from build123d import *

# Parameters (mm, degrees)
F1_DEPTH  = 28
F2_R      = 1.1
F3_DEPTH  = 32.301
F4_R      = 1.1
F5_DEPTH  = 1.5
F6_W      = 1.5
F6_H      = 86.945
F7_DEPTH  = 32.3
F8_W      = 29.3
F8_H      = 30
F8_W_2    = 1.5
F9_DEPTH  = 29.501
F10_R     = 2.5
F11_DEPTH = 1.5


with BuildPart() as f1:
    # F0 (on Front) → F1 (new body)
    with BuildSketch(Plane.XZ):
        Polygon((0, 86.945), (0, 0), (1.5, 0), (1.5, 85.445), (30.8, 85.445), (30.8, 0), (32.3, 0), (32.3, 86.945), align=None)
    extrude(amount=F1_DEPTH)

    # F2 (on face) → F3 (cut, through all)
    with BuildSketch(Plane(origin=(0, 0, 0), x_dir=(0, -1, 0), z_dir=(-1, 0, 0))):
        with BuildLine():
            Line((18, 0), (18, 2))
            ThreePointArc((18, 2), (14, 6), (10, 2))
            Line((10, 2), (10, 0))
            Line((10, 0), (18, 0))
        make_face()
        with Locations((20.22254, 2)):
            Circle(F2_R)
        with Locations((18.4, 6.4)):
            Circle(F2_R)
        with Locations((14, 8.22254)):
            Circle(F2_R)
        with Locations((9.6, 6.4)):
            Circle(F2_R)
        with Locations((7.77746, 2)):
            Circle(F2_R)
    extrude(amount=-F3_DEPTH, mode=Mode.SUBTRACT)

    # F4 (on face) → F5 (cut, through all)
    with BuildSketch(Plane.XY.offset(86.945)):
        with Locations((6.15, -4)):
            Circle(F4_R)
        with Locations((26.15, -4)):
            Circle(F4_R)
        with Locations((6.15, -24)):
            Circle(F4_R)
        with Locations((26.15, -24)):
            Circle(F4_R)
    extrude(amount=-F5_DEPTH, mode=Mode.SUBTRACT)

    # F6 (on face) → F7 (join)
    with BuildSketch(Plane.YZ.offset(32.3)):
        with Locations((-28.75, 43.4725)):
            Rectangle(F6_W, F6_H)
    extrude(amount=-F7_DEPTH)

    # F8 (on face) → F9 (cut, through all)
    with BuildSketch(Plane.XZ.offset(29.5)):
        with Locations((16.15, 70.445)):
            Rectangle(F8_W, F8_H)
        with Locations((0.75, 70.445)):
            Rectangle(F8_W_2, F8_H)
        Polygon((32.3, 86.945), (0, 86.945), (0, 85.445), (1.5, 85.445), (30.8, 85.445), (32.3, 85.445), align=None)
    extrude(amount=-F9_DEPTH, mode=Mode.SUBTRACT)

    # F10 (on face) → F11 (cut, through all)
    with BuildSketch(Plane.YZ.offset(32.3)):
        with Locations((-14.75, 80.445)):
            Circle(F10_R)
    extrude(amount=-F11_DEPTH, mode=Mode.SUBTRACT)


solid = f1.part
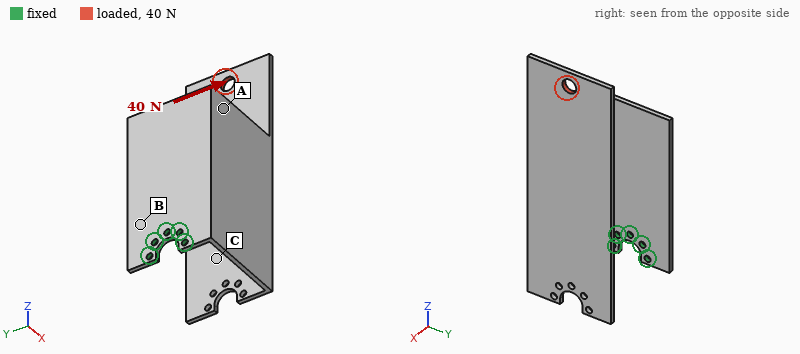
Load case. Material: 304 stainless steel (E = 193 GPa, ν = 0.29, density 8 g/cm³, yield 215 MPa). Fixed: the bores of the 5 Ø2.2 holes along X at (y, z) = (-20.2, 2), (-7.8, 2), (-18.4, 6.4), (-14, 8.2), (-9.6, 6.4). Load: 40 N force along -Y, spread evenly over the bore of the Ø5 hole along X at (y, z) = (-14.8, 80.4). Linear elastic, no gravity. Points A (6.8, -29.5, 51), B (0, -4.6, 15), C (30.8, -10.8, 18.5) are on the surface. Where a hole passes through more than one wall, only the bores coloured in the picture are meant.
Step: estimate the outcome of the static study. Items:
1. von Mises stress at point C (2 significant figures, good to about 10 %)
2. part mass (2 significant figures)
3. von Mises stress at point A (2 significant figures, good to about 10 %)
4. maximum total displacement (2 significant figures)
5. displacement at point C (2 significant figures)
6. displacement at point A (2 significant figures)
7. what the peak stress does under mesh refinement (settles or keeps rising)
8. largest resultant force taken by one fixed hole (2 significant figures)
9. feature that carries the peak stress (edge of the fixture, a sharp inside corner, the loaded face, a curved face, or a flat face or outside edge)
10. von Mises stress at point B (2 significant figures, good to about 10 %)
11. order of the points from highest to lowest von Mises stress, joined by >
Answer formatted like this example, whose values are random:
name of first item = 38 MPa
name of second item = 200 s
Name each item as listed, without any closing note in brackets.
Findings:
von Mises stress at point C = 17 MPa
part mass = 68 g
von Mises stress at point A = 77 MPa
maximum total displacement = 1.1 mm
displacement at point C = 0.47 mm
displacement at point A = 0.22 mm
what the peak stress does under mesh refinement = keeps rising
largest resultant force taken by one fixed hole = 140 N
feature that carries the peak stress = edge of the fixture
von Mises stress at point B = 42 MPa
order of the points from highest to lowest von Mises stress, joined by > = A > B > C
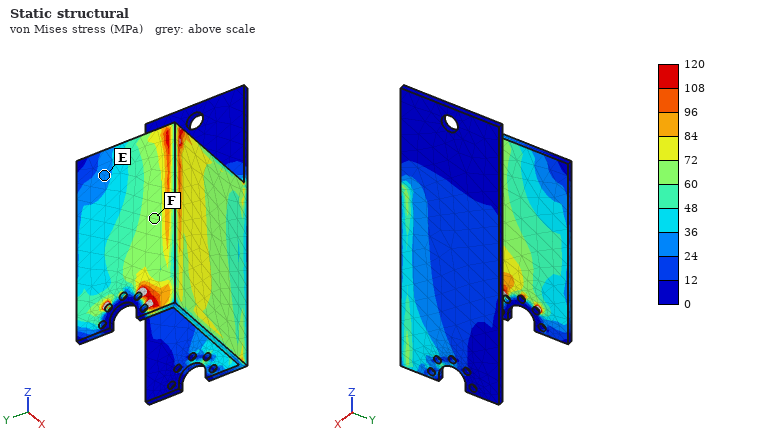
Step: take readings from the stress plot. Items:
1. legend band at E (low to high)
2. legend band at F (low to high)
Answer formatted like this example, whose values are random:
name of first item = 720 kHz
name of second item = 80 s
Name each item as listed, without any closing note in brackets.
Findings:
legend band at E = 24 to 36 MPa
legend band at F = 60 to 72 MPa
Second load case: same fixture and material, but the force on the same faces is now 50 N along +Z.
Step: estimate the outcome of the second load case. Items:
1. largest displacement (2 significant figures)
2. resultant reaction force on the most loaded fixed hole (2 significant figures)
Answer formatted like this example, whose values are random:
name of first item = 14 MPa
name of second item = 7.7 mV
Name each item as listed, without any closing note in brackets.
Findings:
largest displacement = 0.55 mm
resultant reaction force on the most loaded fixed hole = 140 N
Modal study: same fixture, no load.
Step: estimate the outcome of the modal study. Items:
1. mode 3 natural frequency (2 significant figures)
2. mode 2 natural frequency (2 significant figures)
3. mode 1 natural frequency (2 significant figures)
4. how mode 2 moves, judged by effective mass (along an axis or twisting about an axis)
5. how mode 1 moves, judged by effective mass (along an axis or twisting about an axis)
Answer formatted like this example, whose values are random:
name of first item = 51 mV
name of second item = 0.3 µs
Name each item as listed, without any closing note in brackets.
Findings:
mode 3 natural frequency = 530 Hz
mode 2 natural frequency = 260 Hz
mode 1 natural frequency = 230 Hz
how mode 2 moves, judged by effective mass = along X
how mode 1 moves, judged by effective mass = along Y
